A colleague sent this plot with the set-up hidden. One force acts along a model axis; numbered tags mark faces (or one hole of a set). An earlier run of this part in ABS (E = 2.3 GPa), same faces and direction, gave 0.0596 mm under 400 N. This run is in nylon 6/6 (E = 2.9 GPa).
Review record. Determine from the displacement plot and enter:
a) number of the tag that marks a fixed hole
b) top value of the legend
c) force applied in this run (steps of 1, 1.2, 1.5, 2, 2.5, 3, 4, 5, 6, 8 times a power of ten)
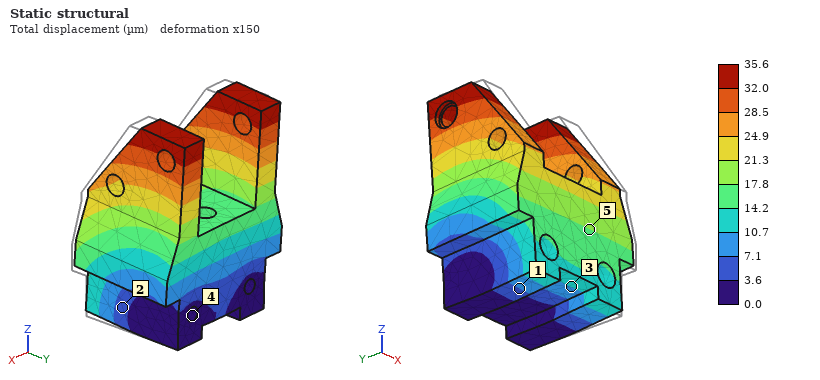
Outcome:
4
35.6 µm
300 N
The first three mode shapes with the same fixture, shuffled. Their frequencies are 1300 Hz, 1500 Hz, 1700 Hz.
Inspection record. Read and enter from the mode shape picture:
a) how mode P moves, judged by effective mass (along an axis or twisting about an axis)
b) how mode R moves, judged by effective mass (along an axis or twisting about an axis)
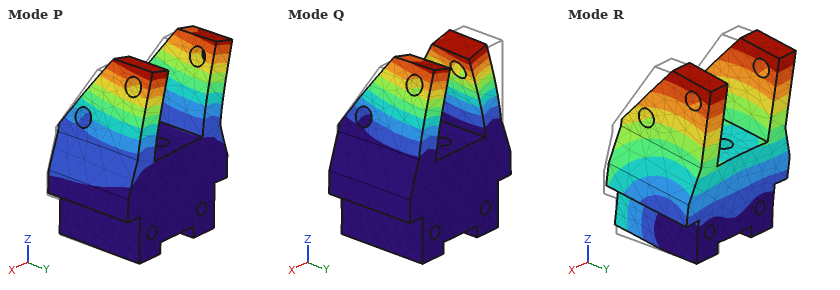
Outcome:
along X
along Y
